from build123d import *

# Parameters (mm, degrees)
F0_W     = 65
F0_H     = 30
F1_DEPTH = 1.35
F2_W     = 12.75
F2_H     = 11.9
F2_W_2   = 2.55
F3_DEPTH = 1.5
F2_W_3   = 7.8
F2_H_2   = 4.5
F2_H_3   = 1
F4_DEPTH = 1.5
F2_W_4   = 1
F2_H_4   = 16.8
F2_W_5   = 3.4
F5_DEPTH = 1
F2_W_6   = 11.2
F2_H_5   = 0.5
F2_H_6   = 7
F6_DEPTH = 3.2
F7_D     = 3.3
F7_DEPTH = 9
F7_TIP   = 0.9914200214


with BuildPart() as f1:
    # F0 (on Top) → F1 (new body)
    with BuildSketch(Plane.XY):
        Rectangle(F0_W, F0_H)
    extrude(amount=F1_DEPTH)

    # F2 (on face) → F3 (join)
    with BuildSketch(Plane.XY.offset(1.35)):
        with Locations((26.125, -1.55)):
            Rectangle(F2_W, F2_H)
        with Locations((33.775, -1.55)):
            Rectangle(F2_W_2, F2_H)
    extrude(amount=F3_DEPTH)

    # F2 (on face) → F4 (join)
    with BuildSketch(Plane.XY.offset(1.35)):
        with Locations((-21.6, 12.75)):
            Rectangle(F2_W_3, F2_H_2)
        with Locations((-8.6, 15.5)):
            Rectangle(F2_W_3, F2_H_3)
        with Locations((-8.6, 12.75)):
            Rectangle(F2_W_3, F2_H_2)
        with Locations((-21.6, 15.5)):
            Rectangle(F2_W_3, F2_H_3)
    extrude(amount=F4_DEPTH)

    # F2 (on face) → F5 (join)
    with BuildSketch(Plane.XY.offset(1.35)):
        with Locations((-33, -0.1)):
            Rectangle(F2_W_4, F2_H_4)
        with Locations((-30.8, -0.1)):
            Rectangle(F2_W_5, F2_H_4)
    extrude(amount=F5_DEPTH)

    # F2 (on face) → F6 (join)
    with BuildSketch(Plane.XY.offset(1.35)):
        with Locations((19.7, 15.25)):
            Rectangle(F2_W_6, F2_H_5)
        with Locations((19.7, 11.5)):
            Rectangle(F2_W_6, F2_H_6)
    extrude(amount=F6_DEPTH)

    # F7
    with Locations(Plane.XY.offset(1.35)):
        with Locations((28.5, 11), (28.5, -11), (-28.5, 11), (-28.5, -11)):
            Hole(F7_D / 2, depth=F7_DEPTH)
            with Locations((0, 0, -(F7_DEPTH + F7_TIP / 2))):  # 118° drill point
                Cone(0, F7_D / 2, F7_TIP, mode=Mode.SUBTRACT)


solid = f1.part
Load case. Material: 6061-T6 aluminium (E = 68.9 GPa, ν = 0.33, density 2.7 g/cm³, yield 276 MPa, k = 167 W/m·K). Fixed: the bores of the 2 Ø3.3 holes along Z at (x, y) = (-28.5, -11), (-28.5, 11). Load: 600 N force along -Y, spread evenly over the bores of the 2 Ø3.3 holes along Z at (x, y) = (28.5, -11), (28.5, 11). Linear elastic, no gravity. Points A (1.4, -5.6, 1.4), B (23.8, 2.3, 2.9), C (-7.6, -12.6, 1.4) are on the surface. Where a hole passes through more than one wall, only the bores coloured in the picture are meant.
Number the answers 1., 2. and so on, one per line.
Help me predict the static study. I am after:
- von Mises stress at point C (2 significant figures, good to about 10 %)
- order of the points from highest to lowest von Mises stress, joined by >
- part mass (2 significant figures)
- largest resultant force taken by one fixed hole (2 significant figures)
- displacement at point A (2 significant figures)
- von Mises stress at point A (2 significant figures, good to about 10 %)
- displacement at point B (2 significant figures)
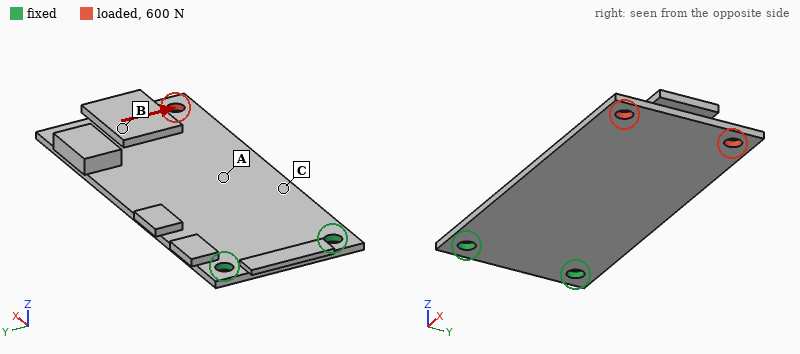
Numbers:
1. 95 MPa
2. C > A > B
3. 9.0 g
4. 1.5 kN
5. 0.11 mm
6. 47 MPa
7. 0.26 mm
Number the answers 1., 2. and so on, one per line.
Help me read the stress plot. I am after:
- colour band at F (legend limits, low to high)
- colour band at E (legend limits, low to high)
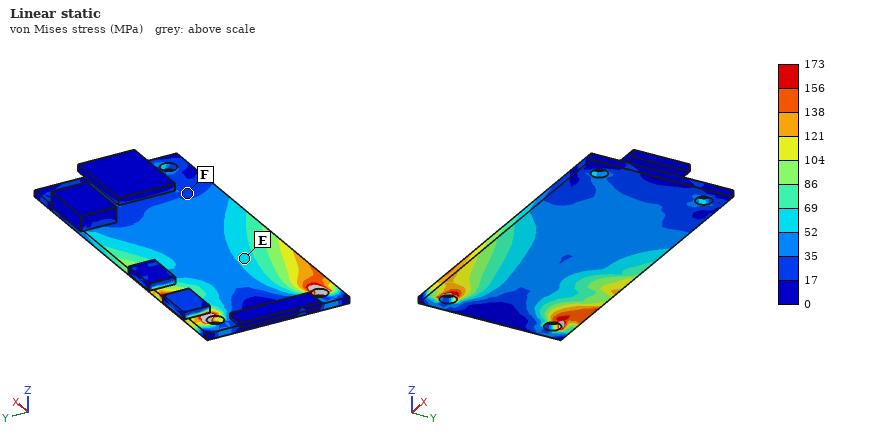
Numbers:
1. 17 to 35 MPa
2. 52 to 69 MPa
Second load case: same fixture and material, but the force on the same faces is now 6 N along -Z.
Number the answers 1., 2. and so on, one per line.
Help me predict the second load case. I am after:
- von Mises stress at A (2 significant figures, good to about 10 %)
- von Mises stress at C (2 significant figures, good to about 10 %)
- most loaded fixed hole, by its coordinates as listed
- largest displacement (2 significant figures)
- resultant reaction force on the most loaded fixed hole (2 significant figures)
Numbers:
1. 16 MPa
2. 21 MPa
3. (-28.5, 11)
4. 0.84 mm
5. 4.6 N
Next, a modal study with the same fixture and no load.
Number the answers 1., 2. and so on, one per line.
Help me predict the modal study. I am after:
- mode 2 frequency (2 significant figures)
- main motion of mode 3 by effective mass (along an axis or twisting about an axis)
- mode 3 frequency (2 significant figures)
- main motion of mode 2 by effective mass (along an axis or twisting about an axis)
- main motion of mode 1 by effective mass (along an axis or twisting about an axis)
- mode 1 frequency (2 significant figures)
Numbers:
1. 1200 Hz
2. along Z
3. 1800 Hz
4. twisting about X
5. along Z
6. 270 Hz
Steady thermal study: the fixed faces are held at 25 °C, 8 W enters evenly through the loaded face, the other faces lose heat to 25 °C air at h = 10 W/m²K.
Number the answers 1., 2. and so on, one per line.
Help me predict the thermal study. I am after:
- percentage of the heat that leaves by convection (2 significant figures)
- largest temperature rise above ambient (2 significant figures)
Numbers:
1. 16 %
2. 61 K
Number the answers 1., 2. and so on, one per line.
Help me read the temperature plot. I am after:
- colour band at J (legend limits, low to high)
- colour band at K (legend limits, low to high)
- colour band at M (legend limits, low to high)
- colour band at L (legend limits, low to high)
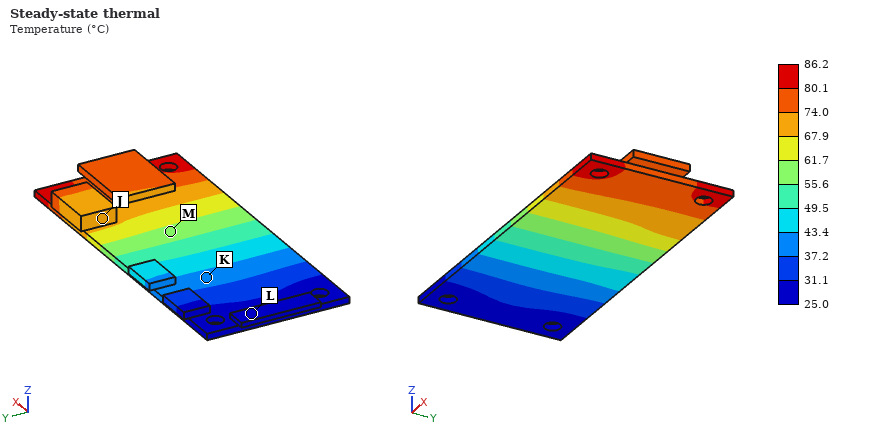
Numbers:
1. 67.9 to 74.0 °C
2. 37.2 to 43.4 °C
3. 55.6 to 61.7 °C
4. 25.0 to 31.1 °C
